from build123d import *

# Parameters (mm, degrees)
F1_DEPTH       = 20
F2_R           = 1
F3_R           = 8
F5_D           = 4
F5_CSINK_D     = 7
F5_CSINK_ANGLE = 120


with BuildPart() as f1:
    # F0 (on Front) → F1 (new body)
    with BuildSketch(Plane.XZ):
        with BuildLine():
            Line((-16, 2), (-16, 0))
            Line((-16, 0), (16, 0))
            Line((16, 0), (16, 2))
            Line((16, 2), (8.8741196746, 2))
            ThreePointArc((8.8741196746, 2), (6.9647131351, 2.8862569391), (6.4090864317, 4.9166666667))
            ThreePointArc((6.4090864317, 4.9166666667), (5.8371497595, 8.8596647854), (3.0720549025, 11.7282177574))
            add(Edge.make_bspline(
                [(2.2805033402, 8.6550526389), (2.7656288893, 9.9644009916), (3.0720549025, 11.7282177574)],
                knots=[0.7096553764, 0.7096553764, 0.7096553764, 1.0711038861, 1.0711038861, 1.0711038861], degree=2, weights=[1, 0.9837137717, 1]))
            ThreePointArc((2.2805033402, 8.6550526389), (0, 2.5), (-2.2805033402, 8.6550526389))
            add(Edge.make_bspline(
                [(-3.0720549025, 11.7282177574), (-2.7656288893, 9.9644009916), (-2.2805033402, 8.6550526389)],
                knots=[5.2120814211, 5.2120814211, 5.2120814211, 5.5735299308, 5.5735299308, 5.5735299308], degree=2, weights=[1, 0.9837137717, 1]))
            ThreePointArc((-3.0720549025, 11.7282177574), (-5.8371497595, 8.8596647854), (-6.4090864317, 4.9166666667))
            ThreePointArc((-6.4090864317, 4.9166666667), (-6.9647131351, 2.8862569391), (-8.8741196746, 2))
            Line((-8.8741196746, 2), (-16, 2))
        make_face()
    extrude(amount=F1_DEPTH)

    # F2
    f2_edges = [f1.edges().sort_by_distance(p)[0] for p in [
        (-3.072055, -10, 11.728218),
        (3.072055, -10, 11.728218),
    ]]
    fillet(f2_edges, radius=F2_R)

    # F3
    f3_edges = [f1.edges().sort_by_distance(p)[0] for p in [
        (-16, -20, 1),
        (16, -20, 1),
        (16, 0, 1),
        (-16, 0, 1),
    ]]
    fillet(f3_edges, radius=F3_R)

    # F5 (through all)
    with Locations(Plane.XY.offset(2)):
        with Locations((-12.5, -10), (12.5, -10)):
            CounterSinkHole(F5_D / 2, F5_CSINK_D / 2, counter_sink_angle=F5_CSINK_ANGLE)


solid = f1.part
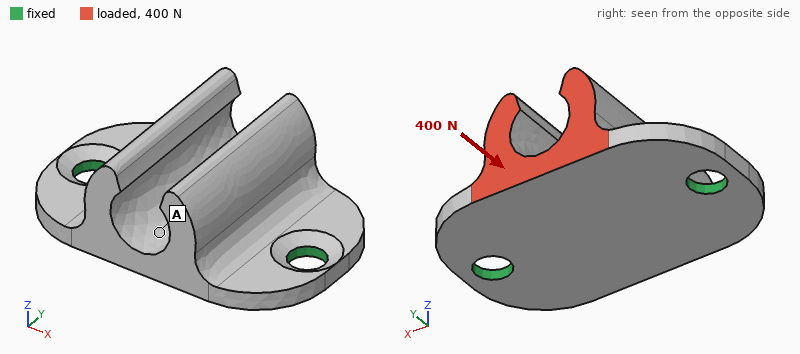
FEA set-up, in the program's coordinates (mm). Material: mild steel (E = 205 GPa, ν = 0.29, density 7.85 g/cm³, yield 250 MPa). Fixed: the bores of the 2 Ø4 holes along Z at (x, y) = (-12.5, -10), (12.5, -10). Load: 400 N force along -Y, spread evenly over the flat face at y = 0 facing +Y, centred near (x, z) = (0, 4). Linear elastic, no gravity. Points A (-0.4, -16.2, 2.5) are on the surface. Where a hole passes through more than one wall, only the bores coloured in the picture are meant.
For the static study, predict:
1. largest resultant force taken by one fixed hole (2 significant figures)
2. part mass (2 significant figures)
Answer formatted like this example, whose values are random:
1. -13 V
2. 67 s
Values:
1. 200 N
2. 19 g
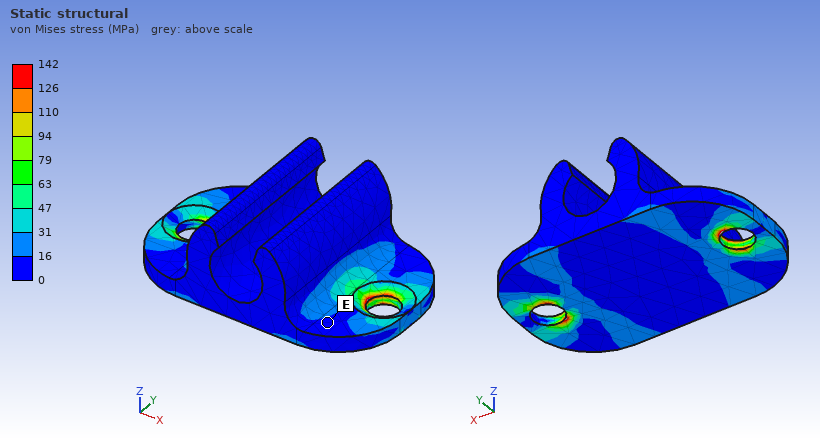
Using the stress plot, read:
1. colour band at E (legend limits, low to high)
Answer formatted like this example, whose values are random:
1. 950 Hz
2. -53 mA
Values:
1. 0 to 16 MPa
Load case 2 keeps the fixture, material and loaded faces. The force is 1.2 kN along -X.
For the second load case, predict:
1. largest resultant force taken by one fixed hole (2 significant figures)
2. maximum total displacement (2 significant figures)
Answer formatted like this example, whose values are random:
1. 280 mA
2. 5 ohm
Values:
1. 780 N
2. 13 µm
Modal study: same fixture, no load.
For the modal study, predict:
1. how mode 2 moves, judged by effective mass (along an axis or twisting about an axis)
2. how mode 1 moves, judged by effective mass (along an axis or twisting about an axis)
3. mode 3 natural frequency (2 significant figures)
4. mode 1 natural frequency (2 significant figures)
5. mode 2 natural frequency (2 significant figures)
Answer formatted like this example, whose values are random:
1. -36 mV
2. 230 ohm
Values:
1. along Z
2. along Y
3. 22 kHz
4. 6300 Hz
5. 11 kHz
